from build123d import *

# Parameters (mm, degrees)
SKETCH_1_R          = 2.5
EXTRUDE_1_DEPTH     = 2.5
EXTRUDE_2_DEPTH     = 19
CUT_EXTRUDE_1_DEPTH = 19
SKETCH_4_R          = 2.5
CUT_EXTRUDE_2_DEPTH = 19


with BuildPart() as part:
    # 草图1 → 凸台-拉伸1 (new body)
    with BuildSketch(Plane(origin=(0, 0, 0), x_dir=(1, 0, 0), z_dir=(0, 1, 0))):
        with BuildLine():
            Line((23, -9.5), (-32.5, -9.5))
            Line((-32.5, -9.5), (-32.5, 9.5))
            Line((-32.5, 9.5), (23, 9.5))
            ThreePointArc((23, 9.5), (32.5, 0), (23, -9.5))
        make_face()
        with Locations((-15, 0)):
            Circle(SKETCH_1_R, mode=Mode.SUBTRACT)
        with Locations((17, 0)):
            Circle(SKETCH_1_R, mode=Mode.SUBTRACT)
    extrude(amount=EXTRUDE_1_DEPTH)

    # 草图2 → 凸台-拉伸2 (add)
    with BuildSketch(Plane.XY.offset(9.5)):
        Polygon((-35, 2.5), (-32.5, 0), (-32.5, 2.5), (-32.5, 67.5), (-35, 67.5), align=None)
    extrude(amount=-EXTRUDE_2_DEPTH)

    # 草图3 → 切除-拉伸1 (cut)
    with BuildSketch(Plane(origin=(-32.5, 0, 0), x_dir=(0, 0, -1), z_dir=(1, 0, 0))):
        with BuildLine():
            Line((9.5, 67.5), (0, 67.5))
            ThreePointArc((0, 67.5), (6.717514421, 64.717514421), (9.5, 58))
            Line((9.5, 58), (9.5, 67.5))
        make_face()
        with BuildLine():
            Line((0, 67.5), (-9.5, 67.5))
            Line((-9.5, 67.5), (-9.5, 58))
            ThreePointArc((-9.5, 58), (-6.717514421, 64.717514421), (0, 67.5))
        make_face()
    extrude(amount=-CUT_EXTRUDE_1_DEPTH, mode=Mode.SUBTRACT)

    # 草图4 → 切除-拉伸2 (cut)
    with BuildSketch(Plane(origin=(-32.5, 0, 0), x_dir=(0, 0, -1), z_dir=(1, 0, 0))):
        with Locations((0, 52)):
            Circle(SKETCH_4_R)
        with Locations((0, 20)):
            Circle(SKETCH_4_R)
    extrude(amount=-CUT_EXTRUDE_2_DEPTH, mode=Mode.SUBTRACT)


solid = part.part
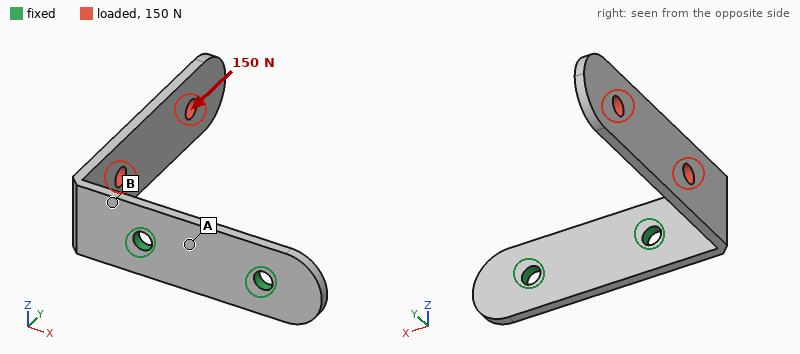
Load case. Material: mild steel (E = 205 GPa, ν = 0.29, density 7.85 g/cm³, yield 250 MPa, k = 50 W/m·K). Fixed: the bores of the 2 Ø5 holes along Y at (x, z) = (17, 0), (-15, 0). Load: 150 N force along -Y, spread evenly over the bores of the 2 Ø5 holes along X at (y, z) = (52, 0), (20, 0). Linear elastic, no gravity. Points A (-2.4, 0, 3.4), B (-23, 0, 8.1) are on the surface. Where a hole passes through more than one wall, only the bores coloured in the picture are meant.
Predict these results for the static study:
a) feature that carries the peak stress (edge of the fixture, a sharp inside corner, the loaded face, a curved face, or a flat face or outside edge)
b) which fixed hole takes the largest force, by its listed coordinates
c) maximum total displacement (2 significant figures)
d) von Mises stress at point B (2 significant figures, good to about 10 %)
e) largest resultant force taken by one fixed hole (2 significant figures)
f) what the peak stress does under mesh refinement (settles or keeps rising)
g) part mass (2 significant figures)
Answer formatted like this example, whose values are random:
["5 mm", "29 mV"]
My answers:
["edge of the fixture", "(-15, 0)", "0.31 mm", "78 MPa", "150 N", "keeps rising", "46 g"]
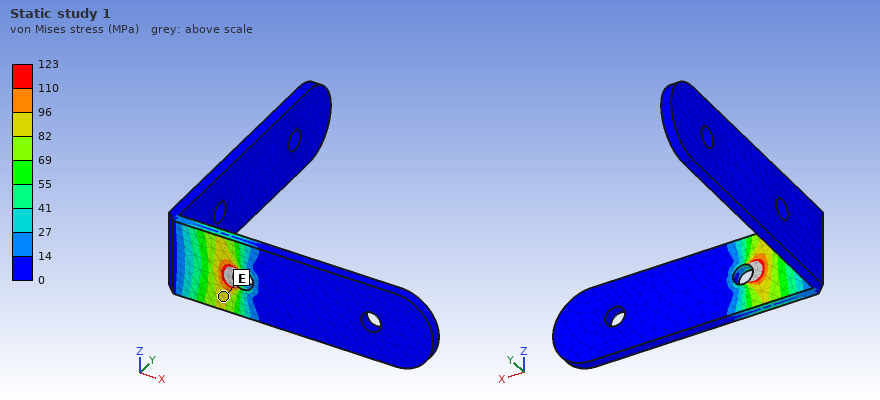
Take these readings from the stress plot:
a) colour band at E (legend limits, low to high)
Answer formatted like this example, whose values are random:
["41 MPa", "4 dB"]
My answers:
["82 to 96 MPa"]
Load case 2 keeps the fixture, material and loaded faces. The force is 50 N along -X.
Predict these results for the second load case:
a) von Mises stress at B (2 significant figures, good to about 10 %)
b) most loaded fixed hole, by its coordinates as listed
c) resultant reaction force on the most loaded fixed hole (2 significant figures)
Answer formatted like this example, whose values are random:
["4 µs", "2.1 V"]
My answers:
["85 MPa", "(-15, 0)", "46 N"]
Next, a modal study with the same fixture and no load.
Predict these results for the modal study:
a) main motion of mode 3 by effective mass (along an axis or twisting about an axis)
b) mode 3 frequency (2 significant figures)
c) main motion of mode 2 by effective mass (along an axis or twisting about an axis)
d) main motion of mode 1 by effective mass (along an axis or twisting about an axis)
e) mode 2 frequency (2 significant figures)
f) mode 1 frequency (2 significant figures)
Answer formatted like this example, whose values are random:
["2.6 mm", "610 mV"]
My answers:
["along Y", "1900 Hz", "along Z", "along X", "610 Hz", "340 Hz"]
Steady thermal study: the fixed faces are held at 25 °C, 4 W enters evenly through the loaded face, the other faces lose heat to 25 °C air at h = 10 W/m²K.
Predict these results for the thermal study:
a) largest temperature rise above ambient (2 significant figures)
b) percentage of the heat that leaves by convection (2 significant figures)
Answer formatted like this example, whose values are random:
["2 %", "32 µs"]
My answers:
["63 K", "35 %"]
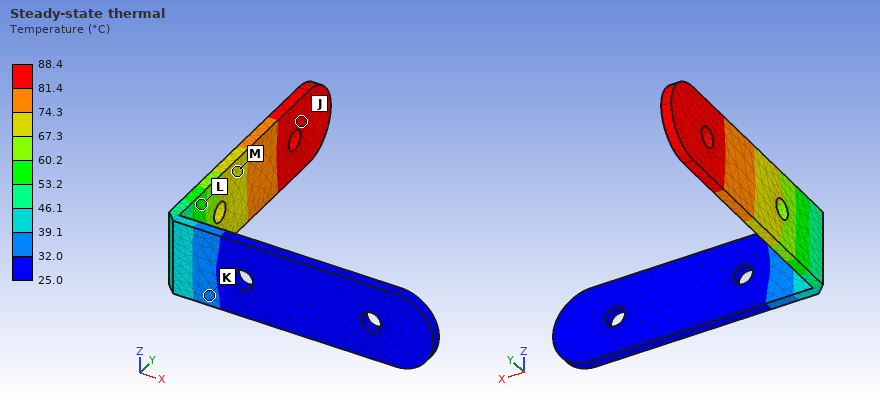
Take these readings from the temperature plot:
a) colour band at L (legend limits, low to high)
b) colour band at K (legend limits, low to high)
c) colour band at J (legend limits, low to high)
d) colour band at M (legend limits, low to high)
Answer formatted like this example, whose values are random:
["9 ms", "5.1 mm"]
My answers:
["53.2 to 60.2 °C", "32.0 to 39.1 °C", "81.4 to 88.4 °C", "67.3 to 74.3 °C"]
